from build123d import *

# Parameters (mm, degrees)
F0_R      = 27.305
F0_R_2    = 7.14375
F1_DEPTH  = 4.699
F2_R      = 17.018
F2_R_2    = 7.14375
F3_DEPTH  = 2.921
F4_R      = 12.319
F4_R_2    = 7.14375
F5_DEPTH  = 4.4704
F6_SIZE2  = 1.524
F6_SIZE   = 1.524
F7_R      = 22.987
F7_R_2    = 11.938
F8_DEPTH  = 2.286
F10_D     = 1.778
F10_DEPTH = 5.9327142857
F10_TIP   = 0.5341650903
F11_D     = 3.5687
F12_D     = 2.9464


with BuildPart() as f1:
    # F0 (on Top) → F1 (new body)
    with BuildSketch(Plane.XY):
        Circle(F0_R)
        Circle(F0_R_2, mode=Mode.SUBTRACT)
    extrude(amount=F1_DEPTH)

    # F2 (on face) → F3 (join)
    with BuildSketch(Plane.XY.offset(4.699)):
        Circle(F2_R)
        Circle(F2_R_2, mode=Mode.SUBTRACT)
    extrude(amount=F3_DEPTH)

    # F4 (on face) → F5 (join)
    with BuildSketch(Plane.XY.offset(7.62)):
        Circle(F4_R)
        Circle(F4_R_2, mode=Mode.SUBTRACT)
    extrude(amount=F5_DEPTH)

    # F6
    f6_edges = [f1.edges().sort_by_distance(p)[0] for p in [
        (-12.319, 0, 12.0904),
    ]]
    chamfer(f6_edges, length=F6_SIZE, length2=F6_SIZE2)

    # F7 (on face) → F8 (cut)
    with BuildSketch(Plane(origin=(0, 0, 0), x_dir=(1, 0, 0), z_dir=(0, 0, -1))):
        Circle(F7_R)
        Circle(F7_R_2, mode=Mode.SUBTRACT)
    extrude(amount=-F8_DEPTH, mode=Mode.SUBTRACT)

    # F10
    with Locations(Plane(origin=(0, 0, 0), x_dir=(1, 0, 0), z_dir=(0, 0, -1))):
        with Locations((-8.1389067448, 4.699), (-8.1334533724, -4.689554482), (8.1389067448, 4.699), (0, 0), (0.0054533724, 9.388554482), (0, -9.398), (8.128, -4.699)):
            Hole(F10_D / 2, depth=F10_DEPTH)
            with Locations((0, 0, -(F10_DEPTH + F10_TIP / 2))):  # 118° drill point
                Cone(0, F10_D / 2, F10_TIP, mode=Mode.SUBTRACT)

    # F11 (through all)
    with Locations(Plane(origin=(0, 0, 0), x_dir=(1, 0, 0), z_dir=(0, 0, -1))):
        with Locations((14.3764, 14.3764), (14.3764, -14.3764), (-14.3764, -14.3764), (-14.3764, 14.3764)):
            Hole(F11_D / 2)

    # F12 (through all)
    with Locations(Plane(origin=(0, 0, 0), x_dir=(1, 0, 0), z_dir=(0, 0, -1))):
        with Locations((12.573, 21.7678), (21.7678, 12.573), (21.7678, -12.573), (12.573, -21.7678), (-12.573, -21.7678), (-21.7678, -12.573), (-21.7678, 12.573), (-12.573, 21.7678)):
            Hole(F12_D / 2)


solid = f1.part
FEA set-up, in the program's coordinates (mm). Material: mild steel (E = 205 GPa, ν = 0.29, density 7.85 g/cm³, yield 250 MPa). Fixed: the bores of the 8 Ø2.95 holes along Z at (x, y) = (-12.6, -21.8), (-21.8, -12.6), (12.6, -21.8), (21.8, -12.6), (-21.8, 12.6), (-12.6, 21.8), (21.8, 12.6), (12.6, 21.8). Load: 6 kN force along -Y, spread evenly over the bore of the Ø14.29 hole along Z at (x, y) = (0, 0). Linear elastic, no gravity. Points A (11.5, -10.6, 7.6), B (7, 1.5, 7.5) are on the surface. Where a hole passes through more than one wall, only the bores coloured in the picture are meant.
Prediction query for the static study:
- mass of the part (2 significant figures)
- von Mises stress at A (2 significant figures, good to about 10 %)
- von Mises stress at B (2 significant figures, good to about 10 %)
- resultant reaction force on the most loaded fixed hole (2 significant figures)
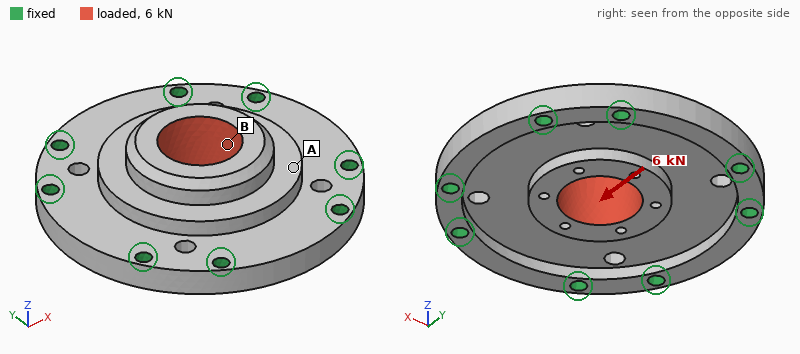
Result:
83 g
8.8 MPa
24 MPa
1000 N
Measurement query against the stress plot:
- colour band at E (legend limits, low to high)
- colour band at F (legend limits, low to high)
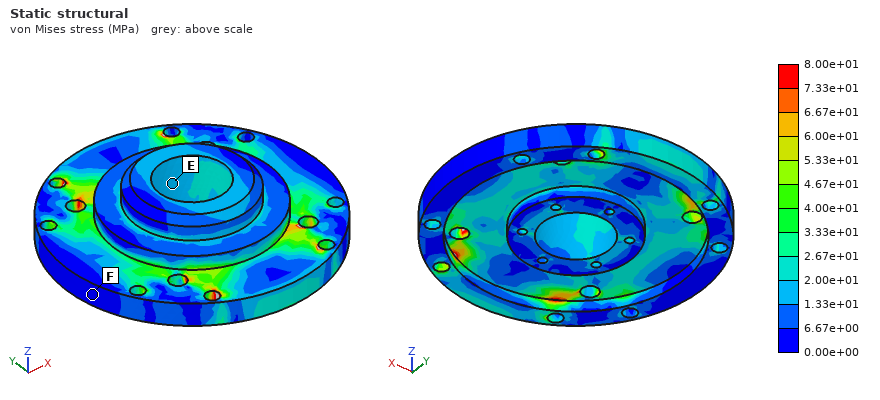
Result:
1.33e+01 to 2.00e+01 MPa
0.00e+00 to 6.67e+00 MPa
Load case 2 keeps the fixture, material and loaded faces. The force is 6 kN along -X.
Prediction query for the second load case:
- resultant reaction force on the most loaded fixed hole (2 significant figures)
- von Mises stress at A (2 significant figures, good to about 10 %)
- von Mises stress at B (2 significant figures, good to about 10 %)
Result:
1.0 kN
9.1 MPa
16 MPa
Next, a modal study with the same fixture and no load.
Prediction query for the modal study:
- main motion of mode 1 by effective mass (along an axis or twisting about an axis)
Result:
along Z
